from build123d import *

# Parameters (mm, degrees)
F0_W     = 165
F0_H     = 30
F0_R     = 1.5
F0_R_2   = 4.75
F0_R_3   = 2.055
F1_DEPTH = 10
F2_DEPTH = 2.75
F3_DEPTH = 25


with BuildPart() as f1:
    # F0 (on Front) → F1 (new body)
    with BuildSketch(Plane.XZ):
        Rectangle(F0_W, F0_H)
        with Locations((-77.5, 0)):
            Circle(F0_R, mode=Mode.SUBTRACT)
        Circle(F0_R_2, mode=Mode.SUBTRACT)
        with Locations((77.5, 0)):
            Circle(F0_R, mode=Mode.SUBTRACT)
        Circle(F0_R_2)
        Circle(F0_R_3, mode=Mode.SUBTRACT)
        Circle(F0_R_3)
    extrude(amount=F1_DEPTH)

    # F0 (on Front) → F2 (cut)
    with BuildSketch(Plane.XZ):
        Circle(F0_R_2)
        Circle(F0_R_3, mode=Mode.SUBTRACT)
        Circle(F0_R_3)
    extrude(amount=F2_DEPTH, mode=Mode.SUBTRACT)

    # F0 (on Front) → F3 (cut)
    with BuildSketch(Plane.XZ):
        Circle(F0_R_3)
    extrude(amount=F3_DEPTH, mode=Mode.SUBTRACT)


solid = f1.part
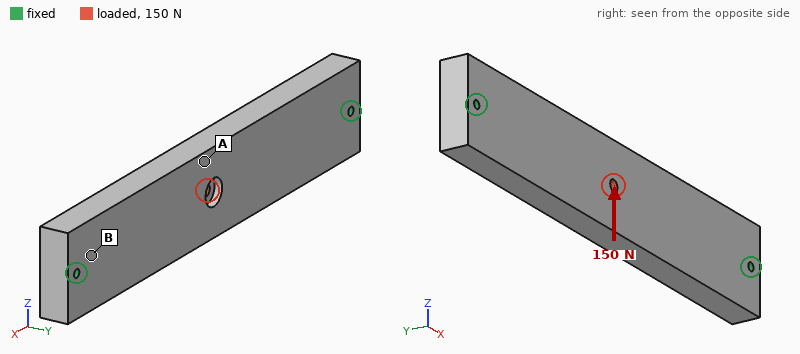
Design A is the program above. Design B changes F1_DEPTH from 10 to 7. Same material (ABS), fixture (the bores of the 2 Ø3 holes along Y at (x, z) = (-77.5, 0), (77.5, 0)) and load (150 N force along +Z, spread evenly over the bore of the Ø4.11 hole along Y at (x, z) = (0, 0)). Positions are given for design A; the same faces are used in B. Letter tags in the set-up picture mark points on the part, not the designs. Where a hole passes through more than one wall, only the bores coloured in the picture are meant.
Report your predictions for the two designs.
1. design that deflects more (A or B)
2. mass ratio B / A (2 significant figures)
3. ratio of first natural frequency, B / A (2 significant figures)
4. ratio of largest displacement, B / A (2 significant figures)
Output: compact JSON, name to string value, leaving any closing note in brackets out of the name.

{"design that deflects more": "B", "mass ratio B / A": "0.70", "ratio of first natural frequency, B / A": "0.73", "ratio of largest displacement, B / A": "1.4"}
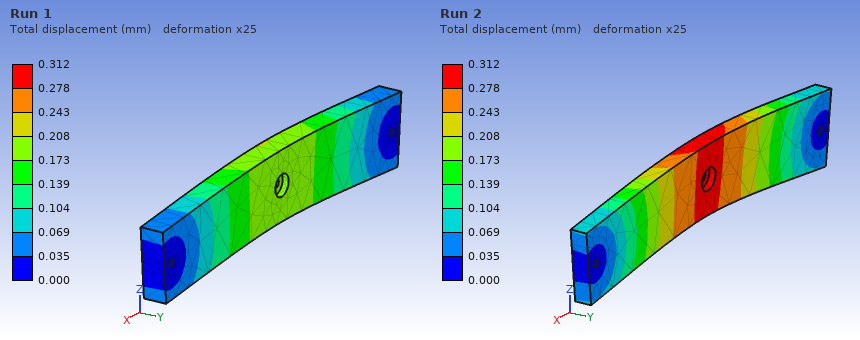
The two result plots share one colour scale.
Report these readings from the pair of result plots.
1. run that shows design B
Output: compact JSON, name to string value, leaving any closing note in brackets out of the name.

{"run that shows design B": "Run 2"}
